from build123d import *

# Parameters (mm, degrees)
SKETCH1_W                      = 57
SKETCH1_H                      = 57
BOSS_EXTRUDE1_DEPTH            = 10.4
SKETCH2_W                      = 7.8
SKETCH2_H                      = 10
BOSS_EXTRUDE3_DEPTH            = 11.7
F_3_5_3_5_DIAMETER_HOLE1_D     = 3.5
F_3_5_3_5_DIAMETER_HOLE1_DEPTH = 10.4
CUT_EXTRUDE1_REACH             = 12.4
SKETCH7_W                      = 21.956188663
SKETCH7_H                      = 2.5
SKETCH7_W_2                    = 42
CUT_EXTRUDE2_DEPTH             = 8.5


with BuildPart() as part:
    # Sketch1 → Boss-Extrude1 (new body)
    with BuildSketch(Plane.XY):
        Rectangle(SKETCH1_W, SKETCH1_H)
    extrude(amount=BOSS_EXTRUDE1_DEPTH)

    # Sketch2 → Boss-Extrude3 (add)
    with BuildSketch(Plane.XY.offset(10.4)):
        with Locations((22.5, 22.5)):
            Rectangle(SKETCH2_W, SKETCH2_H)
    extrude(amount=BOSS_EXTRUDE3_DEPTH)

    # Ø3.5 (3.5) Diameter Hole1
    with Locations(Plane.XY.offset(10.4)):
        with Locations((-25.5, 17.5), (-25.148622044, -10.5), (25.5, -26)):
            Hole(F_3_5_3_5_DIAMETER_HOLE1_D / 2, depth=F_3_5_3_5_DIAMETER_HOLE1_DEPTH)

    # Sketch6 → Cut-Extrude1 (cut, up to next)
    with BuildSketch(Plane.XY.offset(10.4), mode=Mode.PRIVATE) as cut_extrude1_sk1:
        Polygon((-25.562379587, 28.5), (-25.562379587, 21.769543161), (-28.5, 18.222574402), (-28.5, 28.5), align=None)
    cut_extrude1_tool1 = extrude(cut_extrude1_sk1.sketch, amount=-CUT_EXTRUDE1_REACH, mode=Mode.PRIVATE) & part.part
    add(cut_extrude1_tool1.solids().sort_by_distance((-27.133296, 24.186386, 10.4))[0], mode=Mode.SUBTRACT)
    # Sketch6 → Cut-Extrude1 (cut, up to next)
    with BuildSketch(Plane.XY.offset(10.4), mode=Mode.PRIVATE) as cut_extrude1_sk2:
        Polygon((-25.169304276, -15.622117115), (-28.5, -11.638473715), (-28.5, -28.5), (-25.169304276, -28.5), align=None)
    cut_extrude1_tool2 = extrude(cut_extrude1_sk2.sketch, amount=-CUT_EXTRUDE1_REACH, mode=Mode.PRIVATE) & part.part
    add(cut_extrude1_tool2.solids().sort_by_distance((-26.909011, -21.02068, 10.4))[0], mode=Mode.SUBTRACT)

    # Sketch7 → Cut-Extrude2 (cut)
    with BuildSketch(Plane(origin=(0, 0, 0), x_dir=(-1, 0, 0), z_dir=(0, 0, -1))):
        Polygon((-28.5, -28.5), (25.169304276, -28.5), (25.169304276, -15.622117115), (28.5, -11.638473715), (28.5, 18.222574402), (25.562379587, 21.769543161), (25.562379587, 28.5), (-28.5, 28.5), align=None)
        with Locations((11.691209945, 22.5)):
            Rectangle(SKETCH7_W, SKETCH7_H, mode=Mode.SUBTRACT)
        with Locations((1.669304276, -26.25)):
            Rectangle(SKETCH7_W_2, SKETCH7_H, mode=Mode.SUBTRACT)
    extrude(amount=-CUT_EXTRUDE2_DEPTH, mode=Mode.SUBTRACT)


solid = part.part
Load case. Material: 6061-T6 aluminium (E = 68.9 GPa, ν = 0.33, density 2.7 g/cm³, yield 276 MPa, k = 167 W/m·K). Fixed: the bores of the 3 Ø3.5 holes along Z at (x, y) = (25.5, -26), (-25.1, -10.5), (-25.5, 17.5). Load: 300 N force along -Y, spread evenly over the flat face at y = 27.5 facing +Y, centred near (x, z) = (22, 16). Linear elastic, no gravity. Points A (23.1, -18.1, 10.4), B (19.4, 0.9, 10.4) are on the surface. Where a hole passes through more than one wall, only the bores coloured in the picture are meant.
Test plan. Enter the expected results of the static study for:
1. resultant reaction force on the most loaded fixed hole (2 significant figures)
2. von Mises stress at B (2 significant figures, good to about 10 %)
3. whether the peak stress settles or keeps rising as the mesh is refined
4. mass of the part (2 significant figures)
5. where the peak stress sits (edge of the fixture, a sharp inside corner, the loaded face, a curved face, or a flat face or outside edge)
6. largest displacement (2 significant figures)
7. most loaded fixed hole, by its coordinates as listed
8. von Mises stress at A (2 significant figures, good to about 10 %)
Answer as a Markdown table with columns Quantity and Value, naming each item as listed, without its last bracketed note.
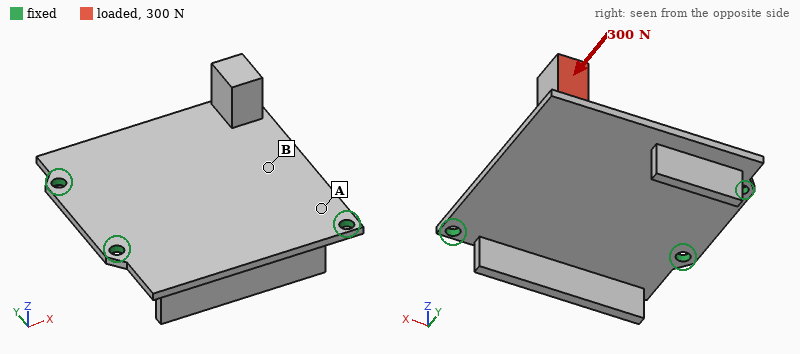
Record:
| Quantity | Value |
|---|---|
| resultant reaction force on the most loaded fixed hole | 220 N |
| von Mises stress at B | 49 MPa |
| whether the peak stress settles or keeps rising as the mesh is refined | keeps rising |
| mass of the part | 22 g |
| where the peak stress sits | edge of the fixture |
| largest displacement | 0.76 mm |
| most loaded fixed hole, by its coordinates as listed | (25.5, -26) |
| von Mises stress at A | 21 MPa |
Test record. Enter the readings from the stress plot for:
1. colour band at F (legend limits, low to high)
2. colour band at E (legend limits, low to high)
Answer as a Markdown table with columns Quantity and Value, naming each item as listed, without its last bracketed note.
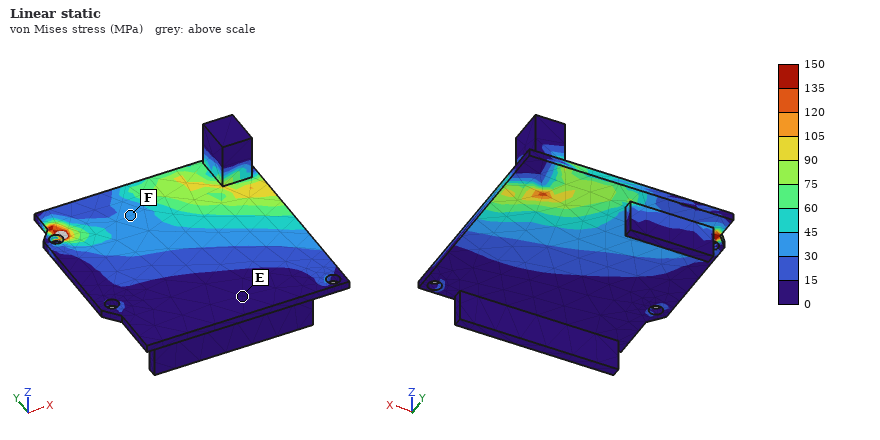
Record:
| Quantity | Value |
|---|---|
| colour band at F | 30 to 45 MPa |
| colour band at E | 0 to 15 MPa |
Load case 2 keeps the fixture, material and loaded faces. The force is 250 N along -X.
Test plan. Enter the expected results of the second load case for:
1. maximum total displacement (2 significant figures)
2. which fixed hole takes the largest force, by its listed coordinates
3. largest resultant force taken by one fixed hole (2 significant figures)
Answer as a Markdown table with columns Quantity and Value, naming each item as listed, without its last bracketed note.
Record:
| Quantity | Value |
|---|---|
| maximum total displacement | 0.65 mm |
| which fixed hole takes the largest force, by its listed coordinates | (-25.5, 17.5) |
| largest resultant force taken by one fixed hole | 180 N |
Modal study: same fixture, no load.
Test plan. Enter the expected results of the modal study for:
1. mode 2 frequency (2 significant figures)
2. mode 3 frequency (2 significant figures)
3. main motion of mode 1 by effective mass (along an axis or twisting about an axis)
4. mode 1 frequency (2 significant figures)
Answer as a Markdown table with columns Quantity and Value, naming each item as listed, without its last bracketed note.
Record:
| Quantity | Value |
|---|---|
| mode 2 frequency | 2700 Hz |
| mode 3 frequency | 2700 Hz |
| main motion of mode 1 by effective mass | along Z |
| mode 1 frequency | 730 Hz |
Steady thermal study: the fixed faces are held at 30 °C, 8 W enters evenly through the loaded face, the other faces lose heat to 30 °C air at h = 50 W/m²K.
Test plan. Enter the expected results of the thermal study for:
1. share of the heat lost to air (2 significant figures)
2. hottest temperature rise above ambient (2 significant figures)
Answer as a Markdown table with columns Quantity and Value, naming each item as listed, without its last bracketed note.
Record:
| Quantity | Value |
|---|---|
| share of the heat lost to air | 35 % |
| hottest temperature rise above ambient | 29 K |
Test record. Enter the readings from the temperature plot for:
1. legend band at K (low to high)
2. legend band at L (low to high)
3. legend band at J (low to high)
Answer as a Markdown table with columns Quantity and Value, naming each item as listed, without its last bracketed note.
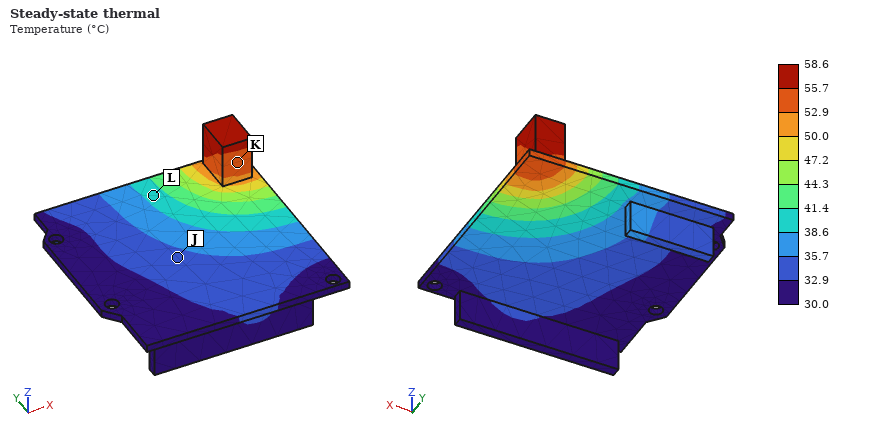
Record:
| Quantity | Value |
|---|---|
| legend band at K | 52.9 to 55.7 °C |
| legend band at L | 38.6 to 41.4 °C |
| legend band at J | 32.9 to 35.7 °C |
